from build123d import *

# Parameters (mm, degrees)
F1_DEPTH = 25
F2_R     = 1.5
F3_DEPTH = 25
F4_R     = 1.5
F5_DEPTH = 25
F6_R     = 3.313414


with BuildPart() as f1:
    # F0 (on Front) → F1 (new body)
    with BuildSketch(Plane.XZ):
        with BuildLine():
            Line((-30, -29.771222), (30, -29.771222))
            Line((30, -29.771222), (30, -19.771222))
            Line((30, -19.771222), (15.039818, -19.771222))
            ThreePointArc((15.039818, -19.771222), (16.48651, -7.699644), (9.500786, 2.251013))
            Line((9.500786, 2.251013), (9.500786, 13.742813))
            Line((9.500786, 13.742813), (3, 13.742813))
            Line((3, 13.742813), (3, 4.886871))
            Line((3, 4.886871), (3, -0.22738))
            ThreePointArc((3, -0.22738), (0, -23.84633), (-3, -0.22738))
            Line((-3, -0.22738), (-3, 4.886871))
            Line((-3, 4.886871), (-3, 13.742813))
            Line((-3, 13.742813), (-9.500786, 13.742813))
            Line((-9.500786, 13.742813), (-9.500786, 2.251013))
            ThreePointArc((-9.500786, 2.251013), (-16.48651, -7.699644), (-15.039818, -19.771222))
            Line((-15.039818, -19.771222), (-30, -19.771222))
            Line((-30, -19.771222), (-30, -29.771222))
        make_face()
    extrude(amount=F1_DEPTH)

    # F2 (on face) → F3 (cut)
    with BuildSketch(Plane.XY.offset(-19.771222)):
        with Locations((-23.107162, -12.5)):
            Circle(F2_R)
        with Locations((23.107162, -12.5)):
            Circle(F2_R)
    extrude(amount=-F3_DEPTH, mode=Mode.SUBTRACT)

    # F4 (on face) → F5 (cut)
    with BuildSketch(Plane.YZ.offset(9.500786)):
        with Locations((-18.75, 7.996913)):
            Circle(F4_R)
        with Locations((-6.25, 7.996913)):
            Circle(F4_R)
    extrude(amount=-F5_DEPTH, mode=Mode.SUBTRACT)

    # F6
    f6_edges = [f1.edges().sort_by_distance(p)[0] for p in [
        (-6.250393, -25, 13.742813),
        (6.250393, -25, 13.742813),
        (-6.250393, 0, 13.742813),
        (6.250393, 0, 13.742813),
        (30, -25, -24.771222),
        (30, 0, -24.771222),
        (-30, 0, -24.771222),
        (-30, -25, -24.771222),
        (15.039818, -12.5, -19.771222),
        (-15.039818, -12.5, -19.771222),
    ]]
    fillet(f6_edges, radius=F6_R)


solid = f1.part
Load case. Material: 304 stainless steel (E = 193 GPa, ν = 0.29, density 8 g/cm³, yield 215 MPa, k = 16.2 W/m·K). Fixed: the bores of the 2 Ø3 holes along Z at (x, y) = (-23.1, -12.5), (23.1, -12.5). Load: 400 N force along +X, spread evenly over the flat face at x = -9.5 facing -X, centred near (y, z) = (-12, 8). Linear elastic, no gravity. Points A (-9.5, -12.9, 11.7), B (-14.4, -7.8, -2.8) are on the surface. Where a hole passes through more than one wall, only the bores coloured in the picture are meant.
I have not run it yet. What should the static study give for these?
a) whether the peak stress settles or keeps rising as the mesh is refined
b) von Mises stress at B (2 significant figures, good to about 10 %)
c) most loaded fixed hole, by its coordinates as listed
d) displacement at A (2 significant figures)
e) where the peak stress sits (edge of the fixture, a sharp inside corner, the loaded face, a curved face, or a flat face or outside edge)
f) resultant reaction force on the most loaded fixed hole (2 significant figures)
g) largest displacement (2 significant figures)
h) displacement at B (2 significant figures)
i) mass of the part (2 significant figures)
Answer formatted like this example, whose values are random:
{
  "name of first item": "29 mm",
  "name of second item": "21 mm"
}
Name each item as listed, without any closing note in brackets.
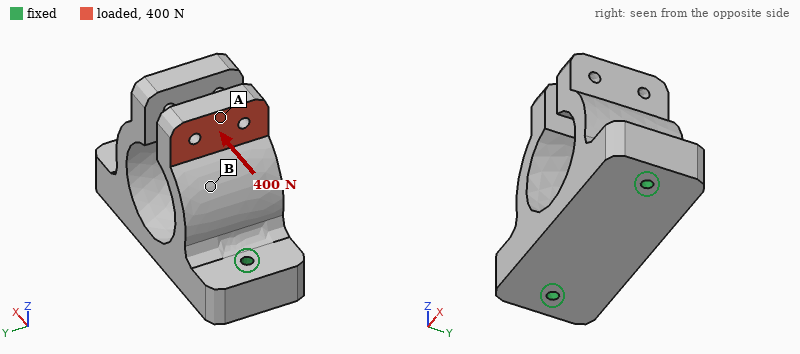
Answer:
{
  "whether the peak stress settles or keeps rising as the mesh is refined": "keeps rising",
  "von Mises stress at B": "40 MPa",
  "most loaded fixed hole, by its coordinates as listed": "(-23.1, -12.5)",
  "displacement at A": "70 µm",
  "where the peak stress sits": "a sharp inside corner",
  "resultant reaction force on the most loaded fixed hole": "650 N",
  "largest displacement": "82 µm",
  "displacement at B": "26 µm",
  "mass of the part": "190 g"
}
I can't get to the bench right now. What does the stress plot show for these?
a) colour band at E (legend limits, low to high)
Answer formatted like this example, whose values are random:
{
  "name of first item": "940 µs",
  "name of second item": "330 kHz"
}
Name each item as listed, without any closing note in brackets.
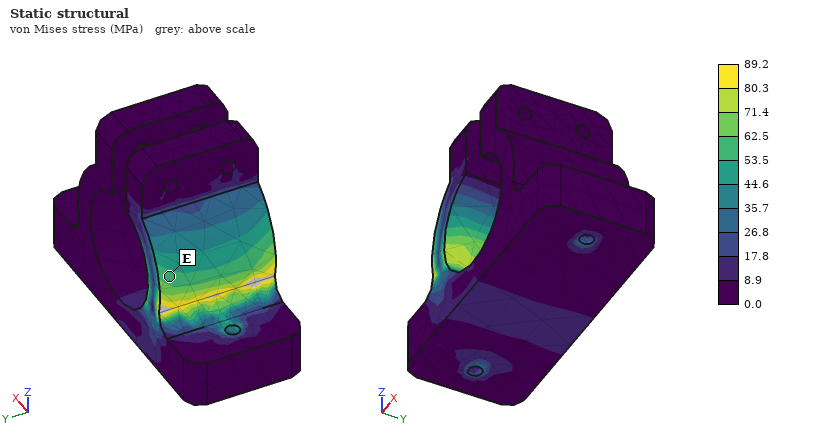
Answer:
{
  "colour band at E": "53.5 to 62.5 MPa"
}
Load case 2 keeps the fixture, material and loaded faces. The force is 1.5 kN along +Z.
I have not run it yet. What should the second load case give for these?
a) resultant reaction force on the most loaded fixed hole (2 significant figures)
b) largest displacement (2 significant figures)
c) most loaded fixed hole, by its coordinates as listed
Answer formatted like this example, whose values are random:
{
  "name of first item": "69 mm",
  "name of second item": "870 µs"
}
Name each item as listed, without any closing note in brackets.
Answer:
{
  "resultant reaction force on the most loaded fixed hole": "1.2 kN",
  "largest displacement": "62 µm",
  "most loaded fixed hole, by its coordinates as listed": "(-23.1, -12.5)"
}
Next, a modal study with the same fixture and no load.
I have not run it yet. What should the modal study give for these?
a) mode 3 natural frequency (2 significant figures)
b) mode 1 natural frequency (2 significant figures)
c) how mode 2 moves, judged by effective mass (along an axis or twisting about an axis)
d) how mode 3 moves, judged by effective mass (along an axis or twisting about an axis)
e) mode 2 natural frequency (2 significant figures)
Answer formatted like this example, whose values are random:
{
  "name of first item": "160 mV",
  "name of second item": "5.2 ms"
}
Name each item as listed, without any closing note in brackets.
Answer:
{
  "mode 3 natural frequency": "5000 Hz",
  "mode 1 natural frequency": "2800 Hz",
  "how mode 2 moves, judged by effective mass": "along X",
  "how mode 3 moves, judged by effective mass": "along Y",
  "mode 2 natural frequency": "3000 Hz"
}
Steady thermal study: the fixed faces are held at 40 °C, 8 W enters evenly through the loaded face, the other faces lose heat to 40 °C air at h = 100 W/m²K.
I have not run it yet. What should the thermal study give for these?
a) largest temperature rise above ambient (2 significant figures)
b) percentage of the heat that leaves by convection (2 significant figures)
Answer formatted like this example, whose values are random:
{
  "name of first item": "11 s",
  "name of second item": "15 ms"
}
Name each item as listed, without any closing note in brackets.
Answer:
{
  "largest temperature rise above ambient": "53 K",
  "percentage of the heat that leaves by convection": "83 %"
}
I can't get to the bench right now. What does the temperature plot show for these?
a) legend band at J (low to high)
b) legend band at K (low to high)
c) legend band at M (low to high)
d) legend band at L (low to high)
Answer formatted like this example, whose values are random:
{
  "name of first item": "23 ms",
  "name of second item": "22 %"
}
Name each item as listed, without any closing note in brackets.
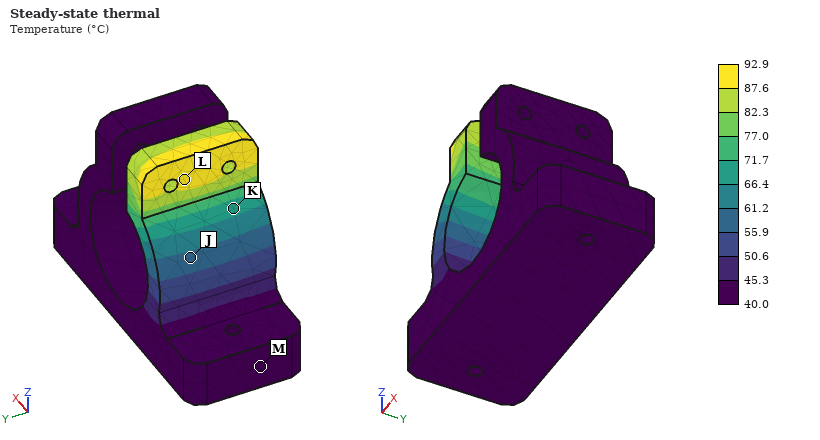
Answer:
{
  "legend band at J": "55.9 to 61.2 °C",
  "legend band at K": "66.4 to 71.7 °C",
  "legend band at M": "40.0 to 45.3 °C",
  "legend band at L": "87.6 to 92.9 °C"
}
